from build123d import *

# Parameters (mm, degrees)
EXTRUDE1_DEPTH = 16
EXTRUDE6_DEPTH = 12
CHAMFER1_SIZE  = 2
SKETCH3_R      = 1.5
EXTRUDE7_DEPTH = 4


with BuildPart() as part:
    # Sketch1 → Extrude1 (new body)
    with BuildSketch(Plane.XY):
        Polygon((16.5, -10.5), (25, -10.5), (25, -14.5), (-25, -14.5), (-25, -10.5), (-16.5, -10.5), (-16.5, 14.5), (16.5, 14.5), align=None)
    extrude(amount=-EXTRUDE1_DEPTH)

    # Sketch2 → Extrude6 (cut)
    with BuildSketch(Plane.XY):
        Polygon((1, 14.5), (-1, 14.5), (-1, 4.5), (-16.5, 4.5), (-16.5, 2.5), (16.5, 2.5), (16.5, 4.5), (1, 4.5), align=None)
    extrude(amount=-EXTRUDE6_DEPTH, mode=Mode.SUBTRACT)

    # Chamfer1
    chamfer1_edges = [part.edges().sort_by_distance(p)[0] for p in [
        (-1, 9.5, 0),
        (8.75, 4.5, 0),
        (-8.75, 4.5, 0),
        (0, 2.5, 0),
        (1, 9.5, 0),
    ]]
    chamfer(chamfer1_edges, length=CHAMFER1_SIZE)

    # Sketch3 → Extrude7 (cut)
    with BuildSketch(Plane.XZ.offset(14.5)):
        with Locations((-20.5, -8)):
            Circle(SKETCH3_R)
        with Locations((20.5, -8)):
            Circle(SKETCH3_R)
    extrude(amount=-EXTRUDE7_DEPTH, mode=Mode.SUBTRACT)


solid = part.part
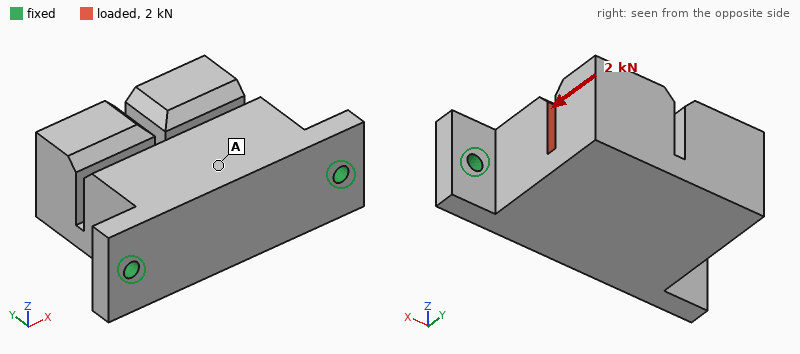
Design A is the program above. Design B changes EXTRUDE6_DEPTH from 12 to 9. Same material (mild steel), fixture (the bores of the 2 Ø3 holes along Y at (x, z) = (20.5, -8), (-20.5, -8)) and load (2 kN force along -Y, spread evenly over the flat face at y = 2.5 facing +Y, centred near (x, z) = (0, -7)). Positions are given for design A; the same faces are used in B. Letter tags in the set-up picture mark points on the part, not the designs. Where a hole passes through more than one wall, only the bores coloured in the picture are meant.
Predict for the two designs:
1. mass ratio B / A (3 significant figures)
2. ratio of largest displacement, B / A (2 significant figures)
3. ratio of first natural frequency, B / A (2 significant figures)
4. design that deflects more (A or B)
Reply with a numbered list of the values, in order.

1. 1.02
2. 2.0
3. 1.0
4. B
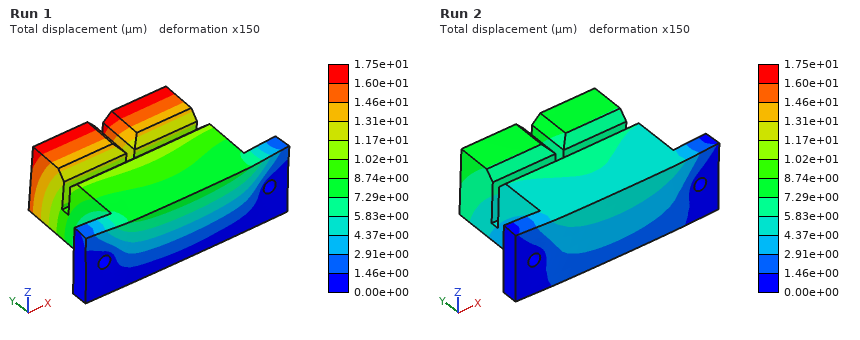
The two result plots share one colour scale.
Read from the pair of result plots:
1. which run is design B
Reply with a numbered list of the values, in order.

1. Run 1
